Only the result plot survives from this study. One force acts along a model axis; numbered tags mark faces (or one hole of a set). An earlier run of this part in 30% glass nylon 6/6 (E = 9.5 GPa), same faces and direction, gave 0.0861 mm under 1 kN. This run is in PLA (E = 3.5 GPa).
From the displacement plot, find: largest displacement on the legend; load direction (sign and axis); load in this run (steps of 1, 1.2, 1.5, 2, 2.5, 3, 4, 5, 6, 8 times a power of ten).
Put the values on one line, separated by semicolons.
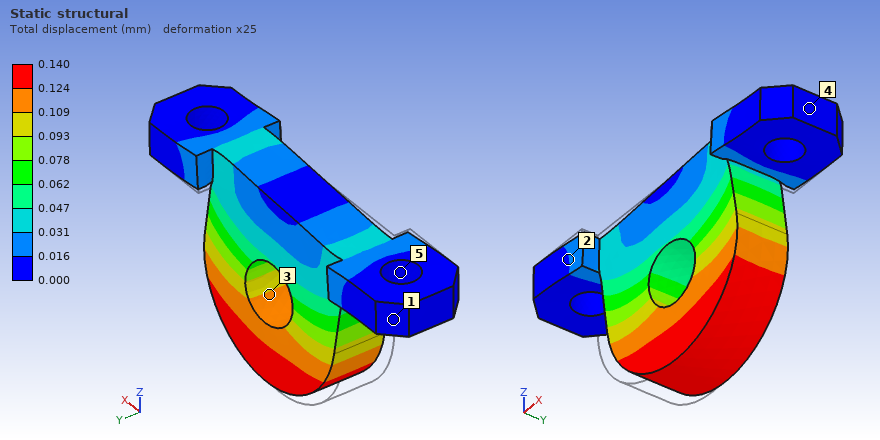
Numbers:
0.140 mm; +X; 600 N
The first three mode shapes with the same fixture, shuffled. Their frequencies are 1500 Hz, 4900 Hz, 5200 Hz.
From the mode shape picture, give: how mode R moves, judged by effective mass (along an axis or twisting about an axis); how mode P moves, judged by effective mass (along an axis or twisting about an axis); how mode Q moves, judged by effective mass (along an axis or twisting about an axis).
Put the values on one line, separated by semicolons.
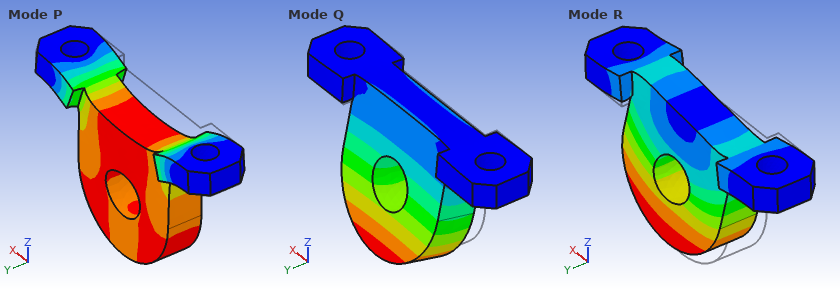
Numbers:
along X; along Z; along Y
